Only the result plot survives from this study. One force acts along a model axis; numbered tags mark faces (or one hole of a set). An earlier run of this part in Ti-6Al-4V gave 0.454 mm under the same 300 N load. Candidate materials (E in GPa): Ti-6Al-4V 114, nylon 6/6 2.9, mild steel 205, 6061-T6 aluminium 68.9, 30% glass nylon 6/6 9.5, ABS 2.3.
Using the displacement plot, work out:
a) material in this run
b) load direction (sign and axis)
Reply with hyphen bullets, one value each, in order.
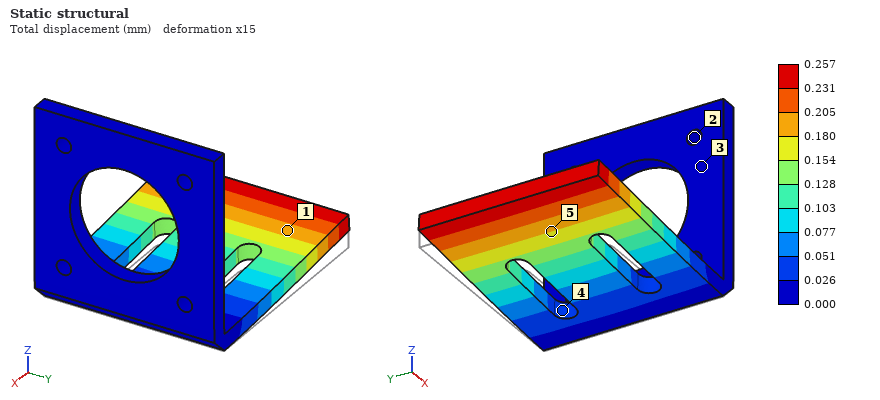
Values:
- mild steel
- +Z
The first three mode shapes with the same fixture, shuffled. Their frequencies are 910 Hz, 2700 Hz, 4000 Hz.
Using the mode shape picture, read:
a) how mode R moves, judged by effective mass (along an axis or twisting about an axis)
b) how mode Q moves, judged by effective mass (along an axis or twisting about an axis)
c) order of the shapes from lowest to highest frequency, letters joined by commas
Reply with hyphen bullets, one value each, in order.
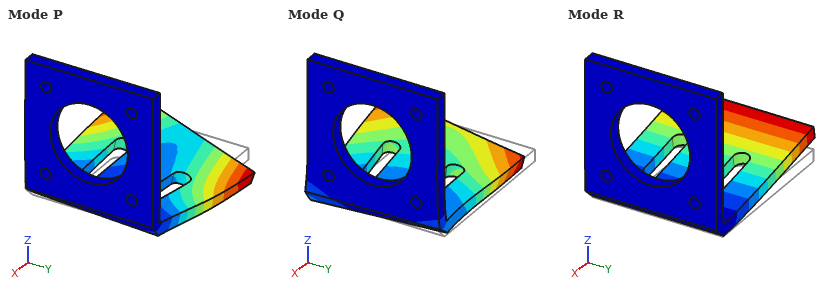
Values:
- along Z
- along Y
- R, P, Q
